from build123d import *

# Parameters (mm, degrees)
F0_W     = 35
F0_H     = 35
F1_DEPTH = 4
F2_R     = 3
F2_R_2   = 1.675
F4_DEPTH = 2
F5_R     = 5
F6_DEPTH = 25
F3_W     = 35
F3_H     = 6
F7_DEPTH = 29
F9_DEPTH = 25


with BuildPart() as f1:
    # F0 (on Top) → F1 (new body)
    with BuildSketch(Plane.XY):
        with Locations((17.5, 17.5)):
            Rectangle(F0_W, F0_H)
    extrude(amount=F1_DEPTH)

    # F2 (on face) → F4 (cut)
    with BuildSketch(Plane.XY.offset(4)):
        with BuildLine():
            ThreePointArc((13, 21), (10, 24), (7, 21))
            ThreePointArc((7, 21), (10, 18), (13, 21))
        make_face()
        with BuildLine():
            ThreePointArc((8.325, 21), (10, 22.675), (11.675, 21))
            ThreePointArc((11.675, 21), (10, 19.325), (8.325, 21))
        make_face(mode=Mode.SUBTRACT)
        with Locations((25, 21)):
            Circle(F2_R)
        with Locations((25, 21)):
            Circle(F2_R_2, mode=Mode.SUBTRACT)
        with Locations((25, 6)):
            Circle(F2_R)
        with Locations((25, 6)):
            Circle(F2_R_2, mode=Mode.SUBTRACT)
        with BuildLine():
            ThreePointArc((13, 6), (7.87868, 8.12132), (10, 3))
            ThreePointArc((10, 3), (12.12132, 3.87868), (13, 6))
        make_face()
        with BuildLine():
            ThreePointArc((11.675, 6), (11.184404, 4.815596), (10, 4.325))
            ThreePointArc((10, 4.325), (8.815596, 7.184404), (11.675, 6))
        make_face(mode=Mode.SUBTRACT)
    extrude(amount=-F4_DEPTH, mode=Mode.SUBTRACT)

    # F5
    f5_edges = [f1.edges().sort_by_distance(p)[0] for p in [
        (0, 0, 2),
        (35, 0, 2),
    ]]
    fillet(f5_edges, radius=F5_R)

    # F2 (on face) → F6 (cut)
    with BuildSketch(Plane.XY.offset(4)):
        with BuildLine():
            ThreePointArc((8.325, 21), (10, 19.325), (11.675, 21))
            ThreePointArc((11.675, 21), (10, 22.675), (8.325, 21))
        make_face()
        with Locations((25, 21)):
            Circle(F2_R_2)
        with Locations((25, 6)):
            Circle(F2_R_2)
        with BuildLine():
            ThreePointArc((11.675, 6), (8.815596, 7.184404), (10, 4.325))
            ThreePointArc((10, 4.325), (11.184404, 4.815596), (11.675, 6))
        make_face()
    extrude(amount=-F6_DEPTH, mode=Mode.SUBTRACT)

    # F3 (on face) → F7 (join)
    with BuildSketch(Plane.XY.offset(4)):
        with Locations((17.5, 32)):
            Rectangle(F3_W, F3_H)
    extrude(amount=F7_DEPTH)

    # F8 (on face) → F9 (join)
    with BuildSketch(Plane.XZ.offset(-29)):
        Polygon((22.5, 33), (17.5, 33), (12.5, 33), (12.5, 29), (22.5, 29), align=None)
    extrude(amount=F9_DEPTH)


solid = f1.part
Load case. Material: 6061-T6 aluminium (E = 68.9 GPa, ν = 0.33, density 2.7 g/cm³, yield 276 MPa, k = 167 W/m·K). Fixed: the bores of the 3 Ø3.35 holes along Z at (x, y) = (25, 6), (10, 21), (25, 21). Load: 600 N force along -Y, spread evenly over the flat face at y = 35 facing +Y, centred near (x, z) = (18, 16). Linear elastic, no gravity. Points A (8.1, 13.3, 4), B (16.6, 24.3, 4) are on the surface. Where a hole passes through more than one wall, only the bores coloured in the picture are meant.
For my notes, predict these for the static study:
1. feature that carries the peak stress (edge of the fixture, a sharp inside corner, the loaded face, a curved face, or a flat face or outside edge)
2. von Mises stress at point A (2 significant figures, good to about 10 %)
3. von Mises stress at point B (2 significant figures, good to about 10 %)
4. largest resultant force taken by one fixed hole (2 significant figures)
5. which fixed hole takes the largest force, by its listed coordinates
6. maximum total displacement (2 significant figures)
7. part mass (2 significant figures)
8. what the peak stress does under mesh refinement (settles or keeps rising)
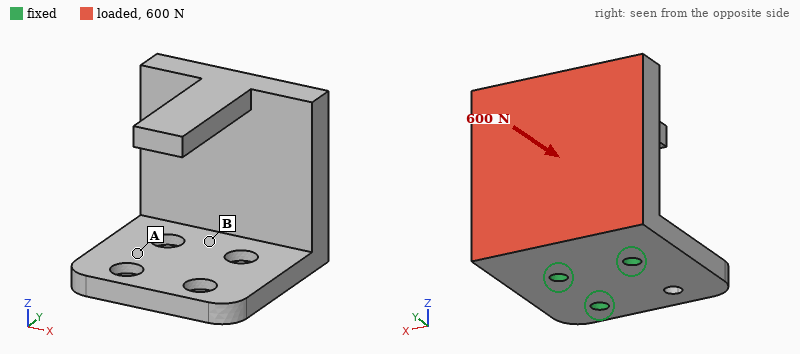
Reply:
edge of the fixture
25 MPa
110 MPa
670 N
(25, 6)
0.41 mm
31 g
keeps rising
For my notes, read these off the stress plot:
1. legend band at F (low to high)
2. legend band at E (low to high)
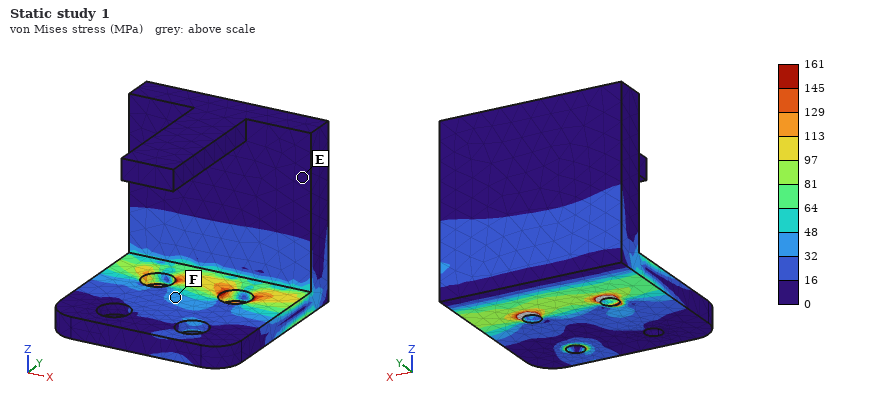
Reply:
32 to 48 MPa
0 to 16 MPa
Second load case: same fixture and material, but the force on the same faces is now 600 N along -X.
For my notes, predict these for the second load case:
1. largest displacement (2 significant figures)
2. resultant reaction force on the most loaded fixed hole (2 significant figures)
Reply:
69 µm
800 N
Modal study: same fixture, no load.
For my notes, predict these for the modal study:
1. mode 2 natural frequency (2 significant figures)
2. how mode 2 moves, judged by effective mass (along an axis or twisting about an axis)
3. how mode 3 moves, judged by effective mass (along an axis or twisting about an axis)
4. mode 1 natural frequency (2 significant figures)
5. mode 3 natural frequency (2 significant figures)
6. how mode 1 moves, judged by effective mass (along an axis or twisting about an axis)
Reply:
3000 Hz
along X
along Z
1500 Hz
4100 Hz
along Y
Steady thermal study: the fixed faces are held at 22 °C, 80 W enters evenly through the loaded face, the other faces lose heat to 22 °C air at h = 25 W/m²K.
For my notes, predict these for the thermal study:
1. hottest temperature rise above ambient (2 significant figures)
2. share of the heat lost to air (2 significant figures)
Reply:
73 K
5.9 %
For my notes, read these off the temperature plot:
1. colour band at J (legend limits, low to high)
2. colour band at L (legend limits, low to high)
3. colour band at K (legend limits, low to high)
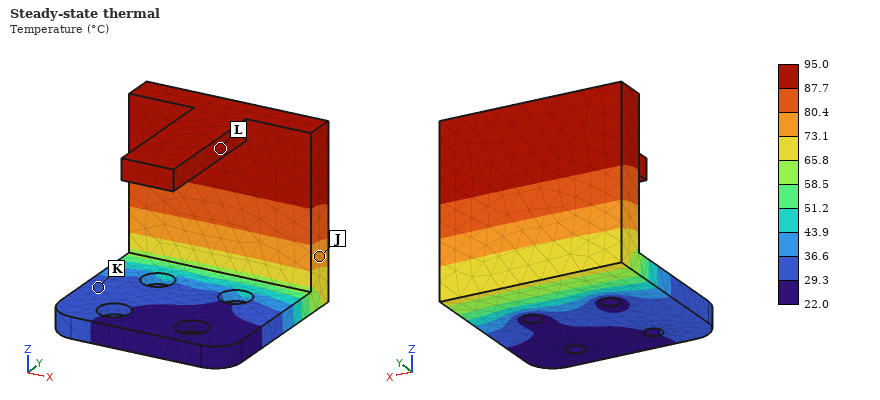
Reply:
73.1 to 80.4 °C
87.7 to 95.0 °C
29.3 to 36.6 °C
